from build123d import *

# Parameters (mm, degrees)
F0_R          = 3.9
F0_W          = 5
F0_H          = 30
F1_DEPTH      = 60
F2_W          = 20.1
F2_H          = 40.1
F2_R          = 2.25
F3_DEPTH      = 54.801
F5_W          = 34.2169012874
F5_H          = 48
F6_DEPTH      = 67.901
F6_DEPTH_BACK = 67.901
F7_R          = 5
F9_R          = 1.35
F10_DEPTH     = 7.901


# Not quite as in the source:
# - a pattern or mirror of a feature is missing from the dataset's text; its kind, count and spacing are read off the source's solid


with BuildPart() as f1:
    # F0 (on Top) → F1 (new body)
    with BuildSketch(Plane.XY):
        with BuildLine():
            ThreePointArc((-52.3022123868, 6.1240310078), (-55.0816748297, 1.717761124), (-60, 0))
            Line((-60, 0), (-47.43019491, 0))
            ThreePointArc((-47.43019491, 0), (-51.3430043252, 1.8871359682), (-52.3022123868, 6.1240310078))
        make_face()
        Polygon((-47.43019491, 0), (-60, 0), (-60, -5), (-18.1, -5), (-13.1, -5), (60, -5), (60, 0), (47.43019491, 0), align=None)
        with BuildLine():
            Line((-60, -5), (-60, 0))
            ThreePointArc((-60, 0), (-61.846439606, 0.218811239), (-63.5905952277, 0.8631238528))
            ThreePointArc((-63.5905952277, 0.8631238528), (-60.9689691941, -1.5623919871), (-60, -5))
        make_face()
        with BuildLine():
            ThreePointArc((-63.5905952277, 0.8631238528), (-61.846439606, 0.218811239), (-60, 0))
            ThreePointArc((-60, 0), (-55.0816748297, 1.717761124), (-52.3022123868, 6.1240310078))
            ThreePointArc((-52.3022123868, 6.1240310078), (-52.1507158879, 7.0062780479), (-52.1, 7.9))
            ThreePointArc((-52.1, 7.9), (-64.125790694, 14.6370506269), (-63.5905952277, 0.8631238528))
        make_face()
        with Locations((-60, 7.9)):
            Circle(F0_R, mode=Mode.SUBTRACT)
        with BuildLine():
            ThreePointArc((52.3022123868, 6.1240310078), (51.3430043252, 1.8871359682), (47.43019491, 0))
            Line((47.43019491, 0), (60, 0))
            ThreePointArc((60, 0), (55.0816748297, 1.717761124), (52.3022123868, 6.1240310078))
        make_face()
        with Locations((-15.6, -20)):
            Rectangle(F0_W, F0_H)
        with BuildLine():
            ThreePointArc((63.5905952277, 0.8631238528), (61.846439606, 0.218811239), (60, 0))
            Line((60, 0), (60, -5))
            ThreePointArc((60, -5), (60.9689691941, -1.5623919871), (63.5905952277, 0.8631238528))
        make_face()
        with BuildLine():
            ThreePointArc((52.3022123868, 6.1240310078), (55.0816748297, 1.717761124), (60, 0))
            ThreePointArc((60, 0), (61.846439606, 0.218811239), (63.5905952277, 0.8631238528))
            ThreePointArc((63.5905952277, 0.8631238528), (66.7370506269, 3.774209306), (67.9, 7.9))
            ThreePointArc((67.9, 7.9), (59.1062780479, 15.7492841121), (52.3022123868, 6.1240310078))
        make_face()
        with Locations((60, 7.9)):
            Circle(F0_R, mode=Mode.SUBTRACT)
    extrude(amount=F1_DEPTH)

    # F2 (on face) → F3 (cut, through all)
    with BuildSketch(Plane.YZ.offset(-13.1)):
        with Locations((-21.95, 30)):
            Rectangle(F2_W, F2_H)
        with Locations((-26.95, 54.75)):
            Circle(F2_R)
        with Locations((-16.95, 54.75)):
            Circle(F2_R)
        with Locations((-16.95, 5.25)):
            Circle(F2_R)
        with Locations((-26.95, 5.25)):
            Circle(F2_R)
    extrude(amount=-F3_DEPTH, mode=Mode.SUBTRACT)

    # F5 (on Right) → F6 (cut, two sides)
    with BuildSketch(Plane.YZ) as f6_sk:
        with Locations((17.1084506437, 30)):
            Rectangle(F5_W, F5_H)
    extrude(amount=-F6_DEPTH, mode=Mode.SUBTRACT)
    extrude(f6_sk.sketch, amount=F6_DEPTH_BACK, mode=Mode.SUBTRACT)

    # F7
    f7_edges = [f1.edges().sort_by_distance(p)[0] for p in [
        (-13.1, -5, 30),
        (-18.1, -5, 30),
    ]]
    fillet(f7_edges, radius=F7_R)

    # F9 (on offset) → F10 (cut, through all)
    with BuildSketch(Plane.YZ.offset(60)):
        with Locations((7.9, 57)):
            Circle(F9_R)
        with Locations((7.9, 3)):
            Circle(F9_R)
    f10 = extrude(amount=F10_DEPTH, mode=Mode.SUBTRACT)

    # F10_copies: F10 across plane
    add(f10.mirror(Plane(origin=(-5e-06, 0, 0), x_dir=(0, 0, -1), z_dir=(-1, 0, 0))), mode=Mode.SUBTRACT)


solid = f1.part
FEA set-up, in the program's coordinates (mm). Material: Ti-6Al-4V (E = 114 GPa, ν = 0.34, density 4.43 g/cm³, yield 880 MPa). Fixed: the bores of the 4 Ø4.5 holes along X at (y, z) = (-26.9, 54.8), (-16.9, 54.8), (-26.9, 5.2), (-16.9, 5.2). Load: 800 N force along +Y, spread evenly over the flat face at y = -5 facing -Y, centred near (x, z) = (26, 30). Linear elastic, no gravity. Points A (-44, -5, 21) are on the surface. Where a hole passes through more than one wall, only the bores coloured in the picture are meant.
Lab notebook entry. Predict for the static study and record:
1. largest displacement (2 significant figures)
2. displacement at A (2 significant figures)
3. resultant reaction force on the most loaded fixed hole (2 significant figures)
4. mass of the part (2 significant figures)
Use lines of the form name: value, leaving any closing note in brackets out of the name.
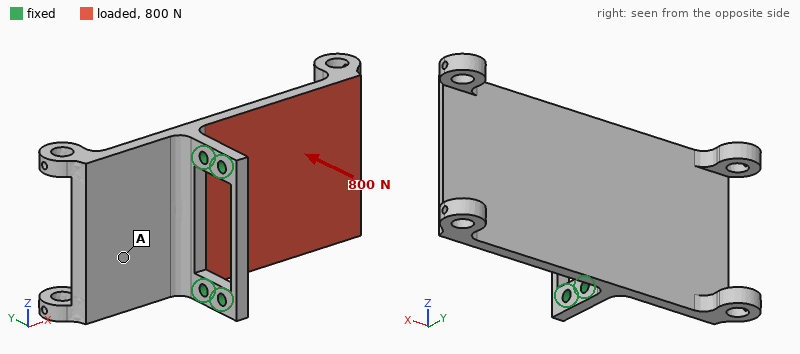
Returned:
largest displacement: 1.6 mm
displacement at A: 0.34 mm
resultant reaction force on the most loaded fixed hole: 540 N
mass of the part: 200 g
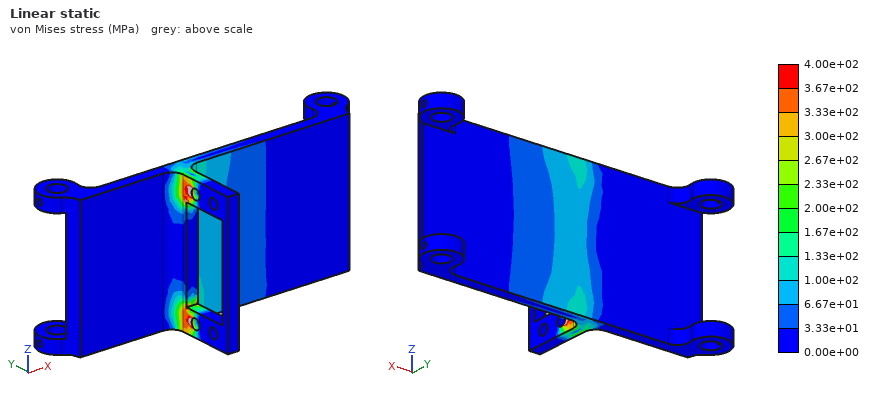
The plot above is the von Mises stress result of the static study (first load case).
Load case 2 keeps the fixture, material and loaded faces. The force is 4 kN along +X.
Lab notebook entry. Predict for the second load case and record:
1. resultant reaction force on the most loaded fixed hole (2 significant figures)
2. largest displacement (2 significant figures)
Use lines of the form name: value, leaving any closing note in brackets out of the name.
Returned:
resultant reaction force on the most loaded fixed hole: 2.2 kN
largest displacement: 0.50 mm
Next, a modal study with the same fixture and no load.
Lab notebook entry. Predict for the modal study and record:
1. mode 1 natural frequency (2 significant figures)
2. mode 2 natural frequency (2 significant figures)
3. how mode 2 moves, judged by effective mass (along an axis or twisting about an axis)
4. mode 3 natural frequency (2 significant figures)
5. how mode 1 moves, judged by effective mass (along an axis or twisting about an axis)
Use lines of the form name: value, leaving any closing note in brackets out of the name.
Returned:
mode 1 natural frequency: 400 Hz
mode 2 natural frequency: 1300 Hz
how mode 2 moves, judged by effective mass: along Y
mode 3 natural frequency: 1500 Hz
how mode 1 moves, judged by effective mass: along Y
